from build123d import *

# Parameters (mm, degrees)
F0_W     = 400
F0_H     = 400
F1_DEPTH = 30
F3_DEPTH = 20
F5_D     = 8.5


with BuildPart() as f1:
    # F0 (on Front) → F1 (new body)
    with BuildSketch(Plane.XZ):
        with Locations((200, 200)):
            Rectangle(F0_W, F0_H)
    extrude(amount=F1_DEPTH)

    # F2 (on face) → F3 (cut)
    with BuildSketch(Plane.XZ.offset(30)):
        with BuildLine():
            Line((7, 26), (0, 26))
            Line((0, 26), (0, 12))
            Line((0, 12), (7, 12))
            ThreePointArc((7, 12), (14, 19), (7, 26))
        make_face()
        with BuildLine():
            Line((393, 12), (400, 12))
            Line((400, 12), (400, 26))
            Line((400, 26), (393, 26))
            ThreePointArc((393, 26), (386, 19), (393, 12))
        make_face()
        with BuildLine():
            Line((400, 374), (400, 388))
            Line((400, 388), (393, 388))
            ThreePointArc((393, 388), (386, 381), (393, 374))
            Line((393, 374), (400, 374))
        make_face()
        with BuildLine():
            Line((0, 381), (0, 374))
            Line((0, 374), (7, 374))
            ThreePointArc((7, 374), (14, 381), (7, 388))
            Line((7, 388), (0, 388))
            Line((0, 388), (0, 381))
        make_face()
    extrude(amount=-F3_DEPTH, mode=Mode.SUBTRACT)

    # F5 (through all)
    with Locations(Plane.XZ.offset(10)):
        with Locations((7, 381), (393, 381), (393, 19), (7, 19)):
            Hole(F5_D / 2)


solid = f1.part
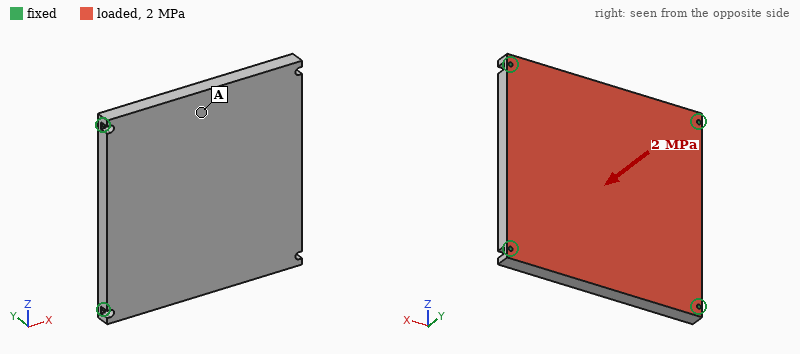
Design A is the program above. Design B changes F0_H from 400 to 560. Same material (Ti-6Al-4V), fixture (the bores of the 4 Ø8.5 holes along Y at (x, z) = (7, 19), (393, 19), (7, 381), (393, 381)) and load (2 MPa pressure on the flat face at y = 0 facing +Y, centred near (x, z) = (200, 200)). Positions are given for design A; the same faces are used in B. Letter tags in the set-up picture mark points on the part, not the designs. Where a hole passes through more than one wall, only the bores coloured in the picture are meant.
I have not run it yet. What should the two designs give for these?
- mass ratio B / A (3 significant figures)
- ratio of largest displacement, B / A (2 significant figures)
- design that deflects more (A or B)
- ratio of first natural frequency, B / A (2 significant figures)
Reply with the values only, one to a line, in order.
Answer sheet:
1.40
0.92
A
1.0
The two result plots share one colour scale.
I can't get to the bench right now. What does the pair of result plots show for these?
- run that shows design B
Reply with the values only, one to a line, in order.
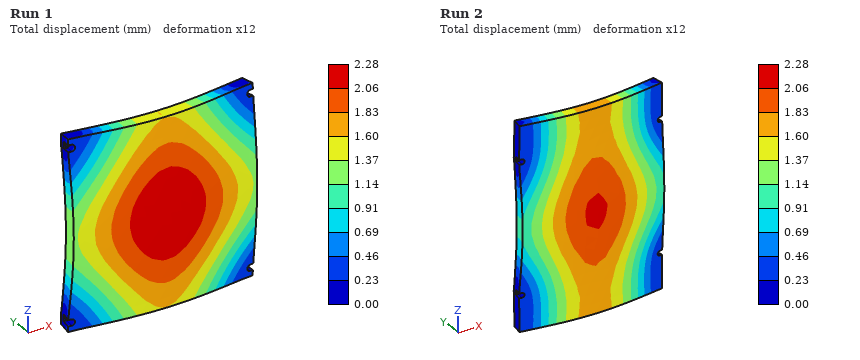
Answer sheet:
Run 2
